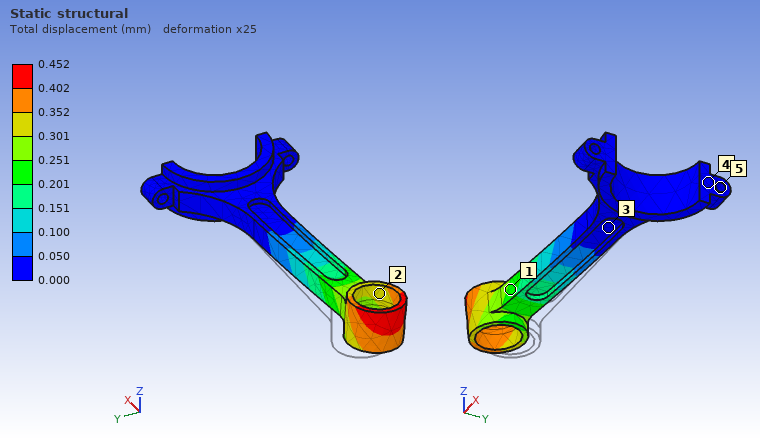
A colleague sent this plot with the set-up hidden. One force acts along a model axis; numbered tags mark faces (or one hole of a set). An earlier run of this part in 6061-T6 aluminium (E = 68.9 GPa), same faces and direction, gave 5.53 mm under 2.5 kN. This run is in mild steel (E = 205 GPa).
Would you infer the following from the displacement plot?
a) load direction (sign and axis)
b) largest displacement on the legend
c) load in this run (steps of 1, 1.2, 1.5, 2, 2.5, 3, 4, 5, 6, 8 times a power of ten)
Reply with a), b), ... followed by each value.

a) -Y
b) 0.452 mm
c) 600 N
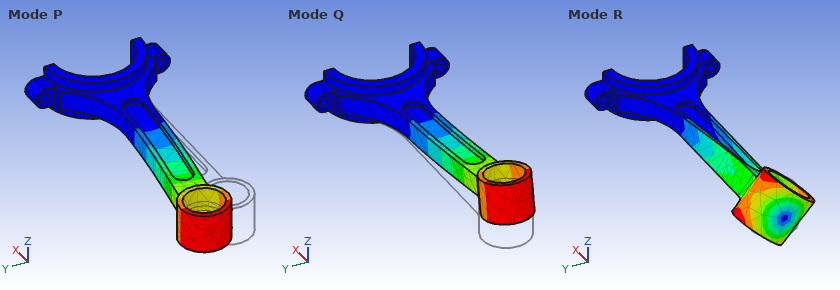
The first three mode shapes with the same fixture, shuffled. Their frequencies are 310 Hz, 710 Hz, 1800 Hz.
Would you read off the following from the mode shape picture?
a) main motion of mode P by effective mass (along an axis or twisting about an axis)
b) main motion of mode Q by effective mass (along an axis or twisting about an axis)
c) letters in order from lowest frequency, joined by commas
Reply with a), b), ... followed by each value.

a) along Y
b) along Z
c) Q, P, R
